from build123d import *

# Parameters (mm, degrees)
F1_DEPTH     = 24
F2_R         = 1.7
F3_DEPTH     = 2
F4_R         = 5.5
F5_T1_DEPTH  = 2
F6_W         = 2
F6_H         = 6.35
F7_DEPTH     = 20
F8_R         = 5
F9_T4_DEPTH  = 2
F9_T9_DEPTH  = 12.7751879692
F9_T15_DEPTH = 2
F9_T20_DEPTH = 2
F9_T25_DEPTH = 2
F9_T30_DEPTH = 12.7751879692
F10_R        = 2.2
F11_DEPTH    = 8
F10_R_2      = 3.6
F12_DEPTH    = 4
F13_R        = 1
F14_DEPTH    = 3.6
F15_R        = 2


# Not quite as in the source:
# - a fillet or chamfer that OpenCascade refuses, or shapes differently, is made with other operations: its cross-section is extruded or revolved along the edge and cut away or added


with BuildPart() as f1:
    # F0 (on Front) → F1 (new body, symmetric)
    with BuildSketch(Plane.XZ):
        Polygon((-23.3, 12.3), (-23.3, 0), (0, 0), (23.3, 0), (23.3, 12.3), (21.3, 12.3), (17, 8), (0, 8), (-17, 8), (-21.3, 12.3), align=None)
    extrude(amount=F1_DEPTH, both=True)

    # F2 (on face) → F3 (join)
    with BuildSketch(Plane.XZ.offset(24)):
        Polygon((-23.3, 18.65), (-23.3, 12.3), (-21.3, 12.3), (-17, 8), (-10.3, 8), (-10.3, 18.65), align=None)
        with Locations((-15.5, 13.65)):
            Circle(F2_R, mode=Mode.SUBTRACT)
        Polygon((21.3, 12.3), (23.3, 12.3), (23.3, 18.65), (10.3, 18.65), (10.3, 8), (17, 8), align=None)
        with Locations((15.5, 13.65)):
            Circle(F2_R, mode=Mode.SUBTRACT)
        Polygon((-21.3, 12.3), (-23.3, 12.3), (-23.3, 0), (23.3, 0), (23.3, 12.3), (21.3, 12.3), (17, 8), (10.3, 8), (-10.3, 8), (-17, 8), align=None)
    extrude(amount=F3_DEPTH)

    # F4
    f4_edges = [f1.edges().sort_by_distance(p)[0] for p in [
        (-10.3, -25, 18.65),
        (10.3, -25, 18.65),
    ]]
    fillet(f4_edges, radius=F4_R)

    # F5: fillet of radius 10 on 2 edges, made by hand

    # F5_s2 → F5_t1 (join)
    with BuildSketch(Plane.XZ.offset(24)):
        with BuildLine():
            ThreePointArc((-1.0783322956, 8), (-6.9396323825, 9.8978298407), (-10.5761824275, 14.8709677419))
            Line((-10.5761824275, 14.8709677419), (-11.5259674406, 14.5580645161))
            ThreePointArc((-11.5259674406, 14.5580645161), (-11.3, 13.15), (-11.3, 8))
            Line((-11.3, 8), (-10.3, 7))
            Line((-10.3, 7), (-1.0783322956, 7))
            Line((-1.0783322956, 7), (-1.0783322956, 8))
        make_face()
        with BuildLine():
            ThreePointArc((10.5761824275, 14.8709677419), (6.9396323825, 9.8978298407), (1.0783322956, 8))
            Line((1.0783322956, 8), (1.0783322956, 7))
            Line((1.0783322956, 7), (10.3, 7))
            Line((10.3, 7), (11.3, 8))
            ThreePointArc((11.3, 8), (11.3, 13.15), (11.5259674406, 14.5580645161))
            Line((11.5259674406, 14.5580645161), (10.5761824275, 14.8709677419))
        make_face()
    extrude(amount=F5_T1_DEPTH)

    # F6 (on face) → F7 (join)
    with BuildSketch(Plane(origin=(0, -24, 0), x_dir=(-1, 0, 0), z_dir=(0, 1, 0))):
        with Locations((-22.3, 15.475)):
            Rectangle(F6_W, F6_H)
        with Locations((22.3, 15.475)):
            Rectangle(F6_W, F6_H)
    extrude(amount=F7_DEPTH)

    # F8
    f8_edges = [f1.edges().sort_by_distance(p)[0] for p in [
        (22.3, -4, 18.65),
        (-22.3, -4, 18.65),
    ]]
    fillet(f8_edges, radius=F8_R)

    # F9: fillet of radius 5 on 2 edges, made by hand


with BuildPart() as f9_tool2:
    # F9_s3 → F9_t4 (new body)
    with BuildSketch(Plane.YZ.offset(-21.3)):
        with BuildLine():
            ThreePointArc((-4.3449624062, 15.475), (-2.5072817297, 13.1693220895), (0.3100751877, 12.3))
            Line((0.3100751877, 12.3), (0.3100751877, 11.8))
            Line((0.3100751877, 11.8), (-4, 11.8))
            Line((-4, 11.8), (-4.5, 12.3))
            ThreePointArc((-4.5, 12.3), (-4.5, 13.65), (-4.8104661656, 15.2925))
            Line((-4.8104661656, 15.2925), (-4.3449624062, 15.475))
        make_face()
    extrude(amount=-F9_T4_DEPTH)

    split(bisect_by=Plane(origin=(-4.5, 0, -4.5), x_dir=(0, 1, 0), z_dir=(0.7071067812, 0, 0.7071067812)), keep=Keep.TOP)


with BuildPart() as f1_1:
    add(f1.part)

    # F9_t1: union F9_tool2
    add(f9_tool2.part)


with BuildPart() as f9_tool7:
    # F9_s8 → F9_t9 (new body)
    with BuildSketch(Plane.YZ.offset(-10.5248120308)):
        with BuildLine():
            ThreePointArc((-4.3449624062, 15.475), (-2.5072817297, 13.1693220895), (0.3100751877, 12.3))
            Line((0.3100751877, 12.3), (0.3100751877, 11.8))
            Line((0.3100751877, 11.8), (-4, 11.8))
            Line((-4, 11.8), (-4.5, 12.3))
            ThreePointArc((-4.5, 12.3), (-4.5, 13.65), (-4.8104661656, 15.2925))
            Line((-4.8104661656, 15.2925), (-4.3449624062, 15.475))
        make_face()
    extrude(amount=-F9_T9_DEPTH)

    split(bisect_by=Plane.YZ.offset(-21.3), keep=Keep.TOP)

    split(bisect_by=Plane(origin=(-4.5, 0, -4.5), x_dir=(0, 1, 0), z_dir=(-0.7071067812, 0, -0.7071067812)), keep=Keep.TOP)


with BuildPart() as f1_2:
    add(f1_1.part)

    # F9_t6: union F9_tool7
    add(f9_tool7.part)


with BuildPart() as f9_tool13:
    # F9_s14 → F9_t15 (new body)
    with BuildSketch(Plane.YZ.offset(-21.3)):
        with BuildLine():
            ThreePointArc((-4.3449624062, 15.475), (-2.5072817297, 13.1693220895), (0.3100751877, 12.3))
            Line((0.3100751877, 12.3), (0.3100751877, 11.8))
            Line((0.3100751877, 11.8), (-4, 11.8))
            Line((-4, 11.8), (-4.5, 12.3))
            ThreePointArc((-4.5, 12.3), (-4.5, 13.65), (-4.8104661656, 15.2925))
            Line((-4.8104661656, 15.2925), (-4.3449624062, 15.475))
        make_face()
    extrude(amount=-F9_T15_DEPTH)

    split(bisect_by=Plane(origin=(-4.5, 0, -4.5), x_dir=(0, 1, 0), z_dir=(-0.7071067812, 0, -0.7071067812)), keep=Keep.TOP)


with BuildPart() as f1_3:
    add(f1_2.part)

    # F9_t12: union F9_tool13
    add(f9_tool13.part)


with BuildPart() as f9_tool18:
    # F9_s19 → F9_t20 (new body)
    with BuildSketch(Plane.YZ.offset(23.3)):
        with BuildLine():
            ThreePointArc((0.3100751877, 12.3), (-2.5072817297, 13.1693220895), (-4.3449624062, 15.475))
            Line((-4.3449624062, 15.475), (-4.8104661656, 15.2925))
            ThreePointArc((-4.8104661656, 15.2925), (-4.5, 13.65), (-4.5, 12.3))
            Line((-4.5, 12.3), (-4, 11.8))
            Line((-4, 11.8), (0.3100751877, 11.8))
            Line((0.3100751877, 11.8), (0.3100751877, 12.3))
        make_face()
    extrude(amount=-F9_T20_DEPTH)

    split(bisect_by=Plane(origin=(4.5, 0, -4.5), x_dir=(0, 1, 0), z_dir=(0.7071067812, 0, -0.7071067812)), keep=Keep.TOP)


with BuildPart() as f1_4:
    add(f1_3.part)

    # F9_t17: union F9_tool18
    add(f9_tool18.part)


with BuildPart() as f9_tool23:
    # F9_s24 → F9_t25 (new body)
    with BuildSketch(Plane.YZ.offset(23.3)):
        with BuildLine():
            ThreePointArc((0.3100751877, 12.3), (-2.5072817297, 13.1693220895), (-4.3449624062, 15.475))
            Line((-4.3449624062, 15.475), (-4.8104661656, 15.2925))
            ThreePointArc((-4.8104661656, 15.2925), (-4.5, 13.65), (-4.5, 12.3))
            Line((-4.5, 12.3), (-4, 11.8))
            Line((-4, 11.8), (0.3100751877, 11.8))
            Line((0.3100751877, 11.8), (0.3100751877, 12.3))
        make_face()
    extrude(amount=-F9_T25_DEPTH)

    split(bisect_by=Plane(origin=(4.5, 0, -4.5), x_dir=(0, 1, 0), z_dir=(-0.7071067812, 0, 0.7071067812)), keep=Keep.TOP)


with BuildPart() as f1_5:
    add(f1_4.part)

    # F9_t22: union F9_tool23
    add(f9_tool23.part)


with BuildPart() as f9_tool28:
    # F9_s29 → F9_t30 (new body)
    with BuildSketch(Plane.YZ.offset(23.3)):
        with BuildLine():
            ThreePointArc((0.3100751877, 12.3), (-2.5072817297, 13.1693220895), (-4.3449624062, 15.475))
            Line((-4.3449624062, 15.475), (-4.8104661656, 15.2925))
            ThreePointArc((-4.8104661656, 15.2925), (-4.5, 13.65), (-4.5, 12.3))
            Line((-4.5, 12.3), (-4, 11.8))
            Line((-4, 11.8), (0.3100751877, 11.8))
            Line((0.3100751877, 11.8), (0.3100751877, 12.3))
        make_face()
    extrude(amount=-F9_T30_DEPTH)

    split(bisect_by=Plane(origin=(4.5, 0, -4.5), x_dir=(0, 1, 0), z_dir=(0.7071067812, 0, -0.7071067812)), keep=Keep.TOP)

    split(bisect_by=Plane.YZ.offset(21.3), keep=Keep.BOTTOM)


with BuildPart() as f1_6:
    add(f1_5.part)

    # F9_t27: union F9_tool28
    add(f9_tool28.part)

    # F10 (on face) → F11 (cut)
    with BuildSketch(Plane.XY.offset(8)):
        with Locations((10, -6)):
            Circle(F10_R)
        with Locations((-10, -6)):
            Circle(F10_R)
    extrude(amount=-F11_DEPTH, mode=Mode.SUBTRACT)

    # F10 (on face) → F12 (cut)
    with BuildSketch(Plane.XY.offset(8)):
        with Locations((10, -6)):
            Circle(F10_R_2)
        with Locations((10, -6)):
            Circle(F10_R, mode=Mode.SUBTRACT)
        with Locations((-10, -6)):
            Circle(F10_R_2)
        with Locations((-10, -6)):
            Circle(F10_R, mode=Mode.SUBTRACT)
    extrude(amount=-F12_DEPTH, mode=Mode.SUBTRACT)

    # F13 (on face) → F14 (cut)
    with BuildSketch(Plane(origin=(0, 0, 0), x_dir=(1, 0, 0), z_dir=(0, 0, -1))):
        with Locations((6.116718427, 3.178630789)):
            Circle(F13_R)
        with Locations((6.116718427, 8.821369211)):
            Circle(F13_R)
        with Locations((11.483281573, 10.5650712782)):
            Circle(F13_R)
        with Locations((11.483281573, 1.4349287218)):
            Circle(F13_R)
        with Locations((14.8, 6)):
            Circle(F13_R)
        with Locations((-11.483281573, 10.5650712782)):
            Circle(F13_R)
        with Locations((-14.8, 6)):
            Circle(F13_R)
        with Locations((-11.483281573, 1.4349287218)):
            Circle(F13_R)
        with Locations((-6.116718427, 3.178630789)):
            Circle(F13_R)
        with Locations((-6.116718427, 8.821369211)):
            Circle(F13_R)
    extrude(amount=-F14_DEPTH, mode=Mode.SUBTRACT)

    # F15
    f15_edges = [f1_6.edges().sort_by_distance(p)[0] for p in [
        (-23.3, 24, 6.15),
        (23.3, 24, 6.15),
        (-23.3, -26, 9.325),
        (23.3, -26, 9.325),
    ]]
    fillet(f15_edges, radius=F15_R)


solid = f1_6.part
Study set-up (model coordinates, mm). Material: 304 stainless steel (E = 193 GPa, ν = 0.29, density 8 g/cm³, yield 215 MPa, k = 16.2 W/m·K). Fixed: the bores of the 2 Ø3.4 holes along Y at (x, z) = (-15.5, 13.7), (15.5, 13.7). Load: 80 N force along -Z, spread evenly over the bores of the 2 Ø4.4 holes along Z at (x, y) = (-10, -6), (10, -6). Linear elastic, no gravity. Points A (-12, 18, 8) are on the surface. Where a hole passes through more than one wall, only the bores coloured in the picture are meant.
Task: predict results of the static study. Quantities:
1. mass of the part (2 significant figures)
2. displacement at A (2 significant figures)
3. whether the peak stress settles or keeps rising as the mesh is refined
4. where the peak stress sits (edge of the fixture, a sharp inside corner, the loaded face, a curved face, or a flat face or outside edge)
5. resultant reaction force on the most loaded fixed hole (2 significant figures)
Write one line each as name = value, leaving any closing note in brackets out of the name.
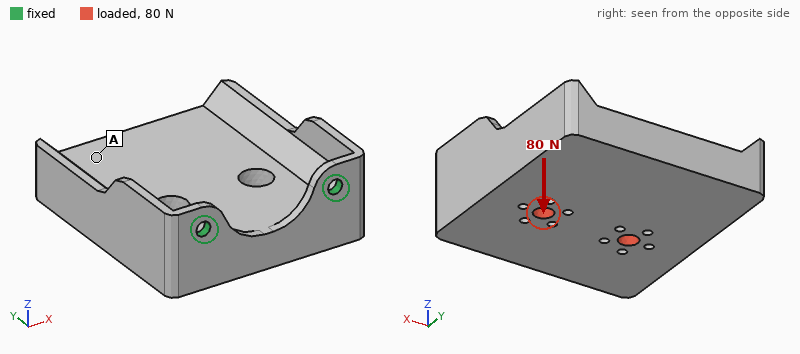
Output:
mass of the part = 170 g
displacement at A = 39 µm
whether the peak stress settles or keeps rising as the mesh is refined = keeps rising
where the peak stress sits = edge of the fixture
resultant reaction force on the most loaded fixed hole = 41 N
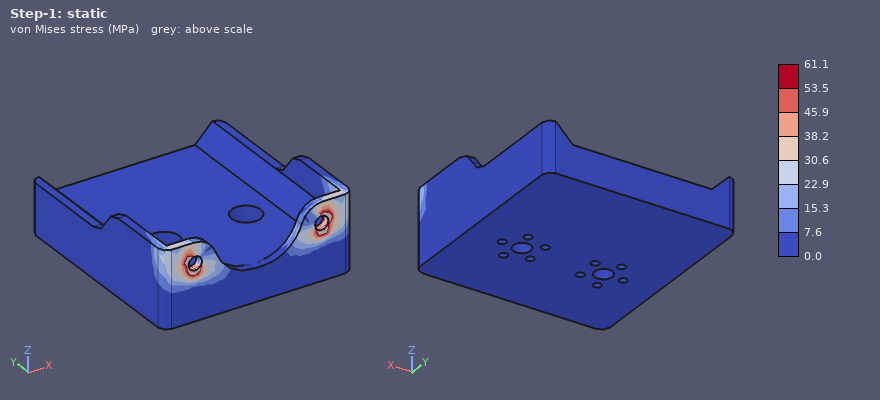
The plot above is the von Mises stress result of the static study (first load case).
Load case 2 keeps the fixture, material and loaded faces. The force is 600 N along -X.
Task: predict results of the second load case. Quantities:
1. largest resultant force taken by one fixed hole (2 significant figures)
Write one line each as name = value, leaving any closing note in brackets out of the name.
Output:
largest resultant force taken by one fixed hole = 480 N
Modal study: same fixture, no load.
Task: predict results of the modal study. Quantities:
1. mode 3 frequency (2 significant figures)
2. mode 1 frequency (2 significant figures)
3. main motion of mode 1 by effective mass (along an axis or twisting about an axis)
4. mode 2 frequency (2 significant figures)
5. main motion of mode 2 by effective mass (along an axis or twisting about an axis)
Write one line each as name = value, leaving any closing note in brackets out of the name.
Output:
mode 3 frequency = 4800 Hz
mode 1 frequency = 560 Hz
main motion of mode 1 by effective mass = along Z
mode 2 frequency = 2500 Hz
main motion of mode 2 by effective mass = along X
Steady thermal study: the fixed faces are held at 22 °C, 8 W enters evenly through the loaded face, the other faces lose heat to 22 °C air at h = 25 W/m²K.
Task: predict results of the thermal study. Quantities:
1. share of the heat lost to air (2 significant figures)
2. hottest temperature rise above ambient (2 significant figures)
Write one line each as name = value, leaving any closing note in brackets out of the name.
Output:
share of the heat lost to air = 62 %
hottest temperature rise above ambient = 43 K
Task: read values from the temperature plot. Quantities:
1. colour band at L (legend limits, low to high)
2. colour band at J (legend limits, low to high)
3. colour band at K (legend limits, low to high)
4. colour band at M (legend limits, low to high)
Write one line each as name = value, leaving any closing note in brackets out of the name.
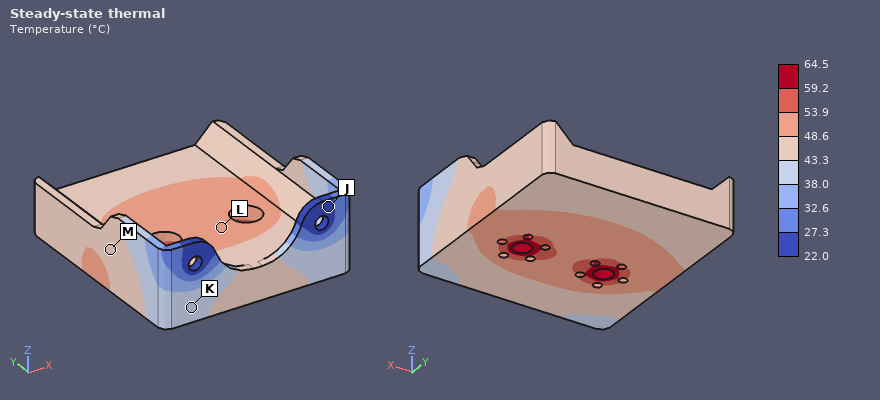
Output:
colour band at L = 48.6 to 53.9 °C
colour band at J = 22.0 to 27.3 °C
colour band at K = 38.0 to 43.3 °C
colour band at M = 43.3 to 48.6 °C
